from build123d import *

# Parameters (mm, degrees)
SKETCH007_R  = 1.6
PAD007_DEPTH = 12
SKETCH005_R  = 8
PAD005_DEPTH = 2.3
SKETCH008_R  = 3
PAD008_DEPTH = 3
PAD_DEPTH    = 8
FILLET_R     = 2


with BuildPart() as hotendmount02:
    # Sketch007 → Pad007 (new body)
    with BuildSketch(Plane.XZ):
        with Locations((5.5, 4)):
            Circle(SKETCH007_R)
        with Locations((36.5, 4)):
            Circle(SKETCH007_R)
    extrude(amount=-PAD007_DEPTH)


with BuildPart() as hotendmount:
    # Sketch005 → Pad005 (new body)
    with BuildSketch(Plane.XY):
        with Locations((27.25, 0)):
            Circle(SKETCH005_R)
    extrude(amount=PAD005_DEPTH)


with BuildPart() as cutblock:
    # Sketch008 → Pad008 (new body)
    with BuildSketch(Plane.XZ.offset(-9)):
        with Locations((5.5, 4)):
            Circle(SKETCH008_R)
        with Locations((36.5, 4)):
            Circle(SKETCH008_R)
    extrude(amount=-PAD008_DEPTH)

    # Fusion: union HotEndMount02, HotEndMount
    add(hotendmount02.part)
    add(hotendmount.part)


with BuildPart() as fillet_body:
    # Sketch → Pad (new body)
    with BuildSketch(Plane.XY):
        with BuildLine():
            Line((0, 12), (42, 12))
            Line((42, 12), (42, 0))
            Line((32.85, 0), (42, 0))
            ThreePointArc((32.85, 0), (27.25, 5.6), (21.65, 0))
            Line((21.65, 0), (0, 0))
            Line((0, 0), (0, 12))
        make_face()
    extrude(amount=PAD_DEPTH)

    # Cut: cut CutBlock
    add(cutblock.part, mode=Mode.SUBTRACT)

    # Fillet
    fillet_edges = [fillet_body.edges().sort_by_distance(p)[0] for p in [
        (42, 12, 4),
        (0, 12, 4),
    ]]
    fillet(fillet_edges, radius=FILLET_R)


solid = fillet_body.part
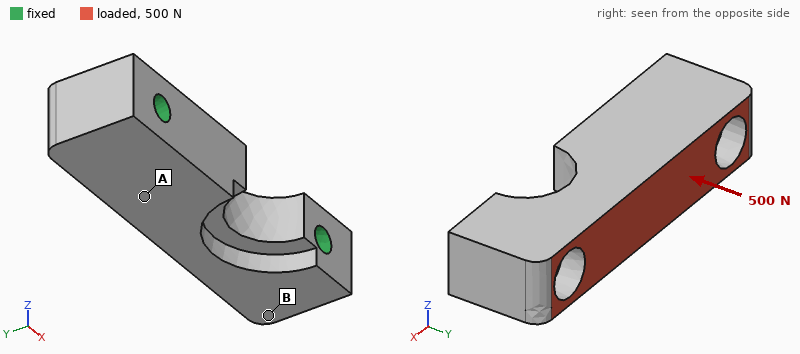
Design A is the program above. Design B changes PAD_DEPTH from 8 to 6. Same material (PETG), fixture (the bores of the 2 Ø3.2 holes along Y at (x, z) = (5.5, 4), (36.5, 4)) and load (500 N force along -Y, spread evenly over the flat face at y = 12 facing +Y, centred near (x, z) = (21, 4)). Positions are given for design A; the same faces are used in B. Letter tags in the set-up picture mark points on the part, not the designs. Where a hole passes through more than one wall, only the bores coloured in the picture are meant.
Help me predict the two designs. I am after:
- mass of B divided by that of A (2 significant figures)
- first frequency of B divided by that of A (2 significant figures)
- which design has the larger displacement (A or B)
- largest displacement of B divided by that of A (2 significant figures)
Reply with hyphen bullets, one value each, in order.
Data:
- 0.72
- 0.89
- B
- 1.5
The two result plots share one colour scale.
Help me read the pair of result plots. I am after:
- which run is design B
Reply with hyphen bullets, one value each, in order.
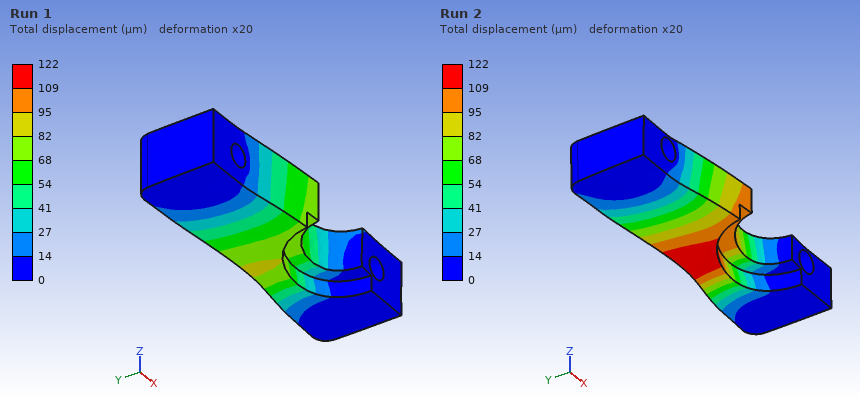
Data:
- Run 2
